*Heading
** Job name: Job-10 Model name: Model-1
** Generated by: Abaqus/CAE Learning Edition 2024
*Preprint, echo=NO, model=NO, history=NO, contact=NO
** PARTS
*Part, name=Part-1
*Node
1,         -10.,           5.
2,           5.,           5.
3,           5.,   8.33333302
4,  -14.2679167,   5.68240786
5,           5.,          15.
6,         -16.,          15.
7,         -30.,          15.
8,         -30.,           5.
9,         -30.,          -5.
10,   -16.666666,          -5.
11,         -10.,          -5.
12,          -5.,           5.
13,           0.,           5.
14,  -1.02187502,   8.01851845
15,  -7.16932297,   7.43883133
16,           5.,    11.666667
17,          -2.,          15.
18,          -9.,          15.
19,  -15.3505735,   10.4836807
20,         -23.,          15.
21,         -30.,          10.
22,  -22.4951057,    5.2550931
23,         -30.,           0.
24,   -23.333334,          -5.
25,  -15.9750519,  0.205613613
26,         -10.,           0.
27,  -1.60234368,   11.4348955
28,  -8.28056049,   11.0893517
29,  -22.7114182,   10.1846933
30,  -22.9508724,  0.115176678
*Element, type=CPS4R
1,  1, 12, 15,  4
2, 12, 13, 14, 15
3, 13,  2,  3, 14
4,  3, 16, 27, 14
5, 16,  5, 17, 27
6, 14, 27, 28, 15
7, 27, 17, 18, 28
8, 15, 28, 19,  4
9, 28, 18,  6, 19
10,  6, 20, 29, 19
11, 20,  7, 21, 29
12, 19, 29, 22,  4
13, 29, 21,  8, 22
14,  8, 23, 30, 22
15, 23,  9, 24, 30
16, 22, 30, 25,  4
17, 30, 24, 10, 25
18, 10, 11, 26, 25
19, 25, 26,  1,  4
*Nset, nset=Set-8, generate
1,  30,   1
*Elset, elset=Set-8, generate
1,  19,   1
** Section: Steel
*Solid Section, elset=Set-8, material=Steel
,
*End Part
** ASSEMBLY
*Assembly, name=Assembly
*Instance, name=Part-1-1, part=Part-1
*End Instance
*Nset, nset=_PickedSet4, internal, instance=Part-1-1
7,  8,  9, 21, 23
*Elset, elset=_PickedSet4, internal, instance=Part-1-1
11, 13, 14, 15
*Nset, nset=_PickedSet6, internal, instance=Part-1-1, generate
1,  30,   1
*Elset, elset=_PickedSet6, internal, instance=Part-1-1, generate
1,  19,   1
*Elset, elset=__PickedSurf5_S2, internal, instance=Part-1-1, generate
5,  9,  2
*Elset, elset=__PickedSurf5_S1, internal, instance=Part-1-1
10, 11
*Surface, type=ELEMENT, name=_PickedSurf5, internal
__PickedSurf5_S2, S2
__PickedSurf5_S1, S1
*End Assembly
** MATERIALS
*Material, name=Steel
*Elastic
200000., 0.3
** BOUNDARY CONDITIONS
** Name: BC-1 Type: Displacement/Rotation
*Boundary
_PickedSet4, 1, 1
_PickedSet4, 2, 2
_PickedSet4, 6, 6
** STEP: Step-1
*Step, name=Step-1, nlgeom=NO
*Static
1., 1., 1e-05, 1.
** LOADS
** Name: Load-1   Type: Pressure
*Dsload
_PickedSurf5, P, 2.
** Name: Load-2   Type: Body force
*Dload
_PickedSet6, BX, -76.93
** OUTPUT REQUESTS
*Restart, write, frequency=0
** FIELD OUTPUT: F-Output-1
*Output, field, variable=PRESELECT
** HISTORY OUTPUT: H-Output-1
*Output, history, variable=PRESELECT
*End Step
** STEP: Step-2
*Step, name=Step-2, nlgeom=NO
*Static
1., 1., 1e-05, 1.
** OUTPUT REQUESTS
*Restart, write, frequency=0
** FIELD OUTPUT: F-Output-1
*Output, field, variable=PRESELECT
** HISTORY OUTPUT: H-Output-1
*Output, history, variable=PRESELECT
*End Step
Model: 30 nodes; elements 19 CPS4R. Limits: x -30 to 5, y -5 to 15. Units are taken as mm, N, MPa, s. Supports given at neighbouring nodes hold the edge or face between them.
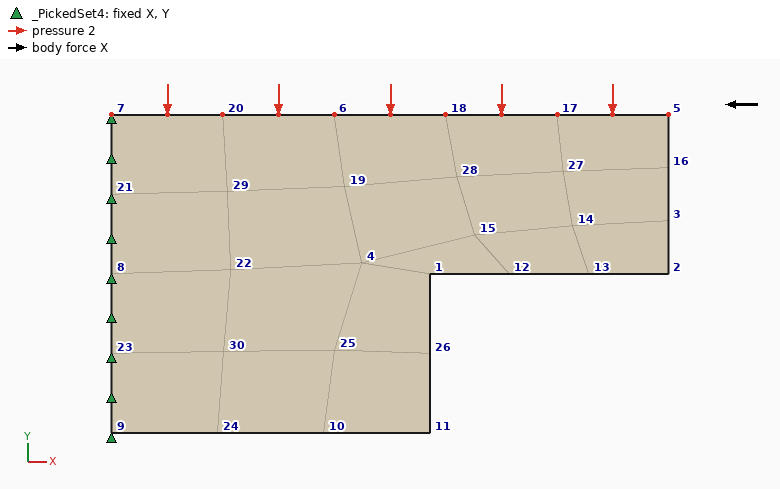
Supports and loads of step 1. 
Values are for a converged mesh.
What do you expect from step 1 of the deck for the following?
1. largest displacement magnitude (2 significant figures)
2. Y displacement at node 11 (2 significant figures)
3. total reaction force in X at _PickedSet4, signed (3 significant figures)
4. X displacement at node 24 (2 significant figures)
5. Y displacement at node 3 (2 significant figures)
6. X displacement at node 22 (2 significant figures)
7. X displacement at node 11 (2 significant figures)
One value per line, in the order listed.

0.32 mm
0.072 mm
42300 N
-0.033 mm
0.20 mm
-0.066 mm
-0.052 mm
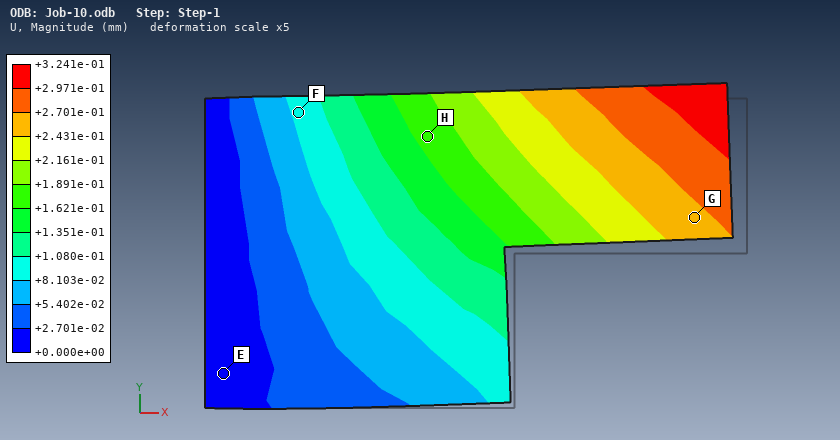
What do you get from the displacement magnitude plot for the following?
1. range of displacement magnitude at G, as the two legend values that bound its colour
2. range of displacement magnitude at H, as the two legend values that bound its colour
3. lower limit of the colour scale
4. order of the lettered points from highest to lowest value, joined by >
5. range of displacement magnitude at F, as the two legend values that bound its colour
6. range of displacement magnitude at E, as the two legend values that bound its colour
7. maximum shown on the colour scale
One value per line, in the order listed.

+2.431e-01 to +2.701e-01 mm
+1.621e-01 to +1.891e-01 mm
+0.000e+00 mm
G > H > F > E
+8.103e-02 to +1.080e-01 mm
+0.000e+00 to +2.701e-02 mm
+3.241e-01 mm
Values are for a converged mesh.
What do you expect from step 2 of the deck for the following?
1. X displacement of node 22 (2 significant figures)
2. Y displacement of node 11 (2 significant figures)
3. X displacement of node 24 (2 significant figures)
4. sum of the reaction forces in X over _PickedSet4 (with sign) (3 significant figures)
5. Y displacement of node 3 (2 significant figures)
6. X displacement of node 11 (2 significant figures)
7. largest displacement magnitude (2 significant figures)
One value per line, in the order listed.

-0.066 mm
0.072 mm
-0.033 mm
42300 N
0.20 mm
-0.052 mm
0.32 mm
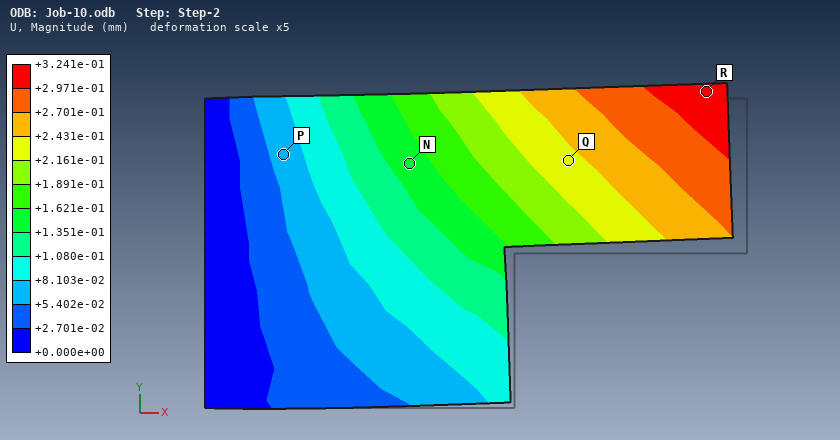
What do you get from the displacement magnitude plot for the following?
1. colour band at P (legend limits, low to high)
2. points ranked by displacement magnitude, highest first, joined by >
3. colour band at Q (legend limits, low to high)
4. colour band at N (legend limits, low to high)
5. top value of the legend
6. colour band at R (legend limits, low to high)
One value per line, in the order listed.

+5.402e-02 to +8.103e-02 mm
R > Q > N > P
+2.161e-01 to +2.431e-01 mm
+1.351e-01 to +1.621e-01 mm
+3.241e-01 mm
+2.971e-01 to +3.241e-01 mm
